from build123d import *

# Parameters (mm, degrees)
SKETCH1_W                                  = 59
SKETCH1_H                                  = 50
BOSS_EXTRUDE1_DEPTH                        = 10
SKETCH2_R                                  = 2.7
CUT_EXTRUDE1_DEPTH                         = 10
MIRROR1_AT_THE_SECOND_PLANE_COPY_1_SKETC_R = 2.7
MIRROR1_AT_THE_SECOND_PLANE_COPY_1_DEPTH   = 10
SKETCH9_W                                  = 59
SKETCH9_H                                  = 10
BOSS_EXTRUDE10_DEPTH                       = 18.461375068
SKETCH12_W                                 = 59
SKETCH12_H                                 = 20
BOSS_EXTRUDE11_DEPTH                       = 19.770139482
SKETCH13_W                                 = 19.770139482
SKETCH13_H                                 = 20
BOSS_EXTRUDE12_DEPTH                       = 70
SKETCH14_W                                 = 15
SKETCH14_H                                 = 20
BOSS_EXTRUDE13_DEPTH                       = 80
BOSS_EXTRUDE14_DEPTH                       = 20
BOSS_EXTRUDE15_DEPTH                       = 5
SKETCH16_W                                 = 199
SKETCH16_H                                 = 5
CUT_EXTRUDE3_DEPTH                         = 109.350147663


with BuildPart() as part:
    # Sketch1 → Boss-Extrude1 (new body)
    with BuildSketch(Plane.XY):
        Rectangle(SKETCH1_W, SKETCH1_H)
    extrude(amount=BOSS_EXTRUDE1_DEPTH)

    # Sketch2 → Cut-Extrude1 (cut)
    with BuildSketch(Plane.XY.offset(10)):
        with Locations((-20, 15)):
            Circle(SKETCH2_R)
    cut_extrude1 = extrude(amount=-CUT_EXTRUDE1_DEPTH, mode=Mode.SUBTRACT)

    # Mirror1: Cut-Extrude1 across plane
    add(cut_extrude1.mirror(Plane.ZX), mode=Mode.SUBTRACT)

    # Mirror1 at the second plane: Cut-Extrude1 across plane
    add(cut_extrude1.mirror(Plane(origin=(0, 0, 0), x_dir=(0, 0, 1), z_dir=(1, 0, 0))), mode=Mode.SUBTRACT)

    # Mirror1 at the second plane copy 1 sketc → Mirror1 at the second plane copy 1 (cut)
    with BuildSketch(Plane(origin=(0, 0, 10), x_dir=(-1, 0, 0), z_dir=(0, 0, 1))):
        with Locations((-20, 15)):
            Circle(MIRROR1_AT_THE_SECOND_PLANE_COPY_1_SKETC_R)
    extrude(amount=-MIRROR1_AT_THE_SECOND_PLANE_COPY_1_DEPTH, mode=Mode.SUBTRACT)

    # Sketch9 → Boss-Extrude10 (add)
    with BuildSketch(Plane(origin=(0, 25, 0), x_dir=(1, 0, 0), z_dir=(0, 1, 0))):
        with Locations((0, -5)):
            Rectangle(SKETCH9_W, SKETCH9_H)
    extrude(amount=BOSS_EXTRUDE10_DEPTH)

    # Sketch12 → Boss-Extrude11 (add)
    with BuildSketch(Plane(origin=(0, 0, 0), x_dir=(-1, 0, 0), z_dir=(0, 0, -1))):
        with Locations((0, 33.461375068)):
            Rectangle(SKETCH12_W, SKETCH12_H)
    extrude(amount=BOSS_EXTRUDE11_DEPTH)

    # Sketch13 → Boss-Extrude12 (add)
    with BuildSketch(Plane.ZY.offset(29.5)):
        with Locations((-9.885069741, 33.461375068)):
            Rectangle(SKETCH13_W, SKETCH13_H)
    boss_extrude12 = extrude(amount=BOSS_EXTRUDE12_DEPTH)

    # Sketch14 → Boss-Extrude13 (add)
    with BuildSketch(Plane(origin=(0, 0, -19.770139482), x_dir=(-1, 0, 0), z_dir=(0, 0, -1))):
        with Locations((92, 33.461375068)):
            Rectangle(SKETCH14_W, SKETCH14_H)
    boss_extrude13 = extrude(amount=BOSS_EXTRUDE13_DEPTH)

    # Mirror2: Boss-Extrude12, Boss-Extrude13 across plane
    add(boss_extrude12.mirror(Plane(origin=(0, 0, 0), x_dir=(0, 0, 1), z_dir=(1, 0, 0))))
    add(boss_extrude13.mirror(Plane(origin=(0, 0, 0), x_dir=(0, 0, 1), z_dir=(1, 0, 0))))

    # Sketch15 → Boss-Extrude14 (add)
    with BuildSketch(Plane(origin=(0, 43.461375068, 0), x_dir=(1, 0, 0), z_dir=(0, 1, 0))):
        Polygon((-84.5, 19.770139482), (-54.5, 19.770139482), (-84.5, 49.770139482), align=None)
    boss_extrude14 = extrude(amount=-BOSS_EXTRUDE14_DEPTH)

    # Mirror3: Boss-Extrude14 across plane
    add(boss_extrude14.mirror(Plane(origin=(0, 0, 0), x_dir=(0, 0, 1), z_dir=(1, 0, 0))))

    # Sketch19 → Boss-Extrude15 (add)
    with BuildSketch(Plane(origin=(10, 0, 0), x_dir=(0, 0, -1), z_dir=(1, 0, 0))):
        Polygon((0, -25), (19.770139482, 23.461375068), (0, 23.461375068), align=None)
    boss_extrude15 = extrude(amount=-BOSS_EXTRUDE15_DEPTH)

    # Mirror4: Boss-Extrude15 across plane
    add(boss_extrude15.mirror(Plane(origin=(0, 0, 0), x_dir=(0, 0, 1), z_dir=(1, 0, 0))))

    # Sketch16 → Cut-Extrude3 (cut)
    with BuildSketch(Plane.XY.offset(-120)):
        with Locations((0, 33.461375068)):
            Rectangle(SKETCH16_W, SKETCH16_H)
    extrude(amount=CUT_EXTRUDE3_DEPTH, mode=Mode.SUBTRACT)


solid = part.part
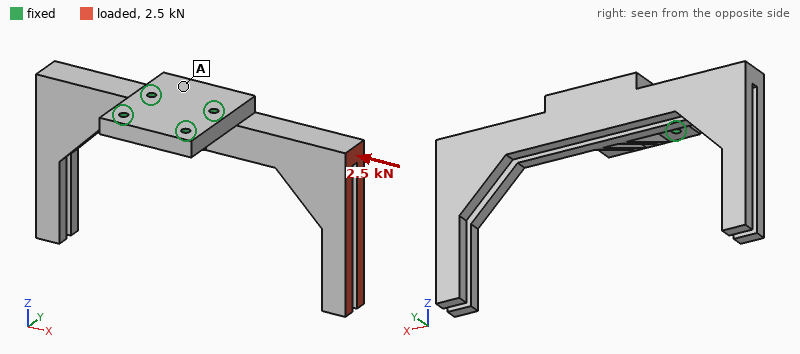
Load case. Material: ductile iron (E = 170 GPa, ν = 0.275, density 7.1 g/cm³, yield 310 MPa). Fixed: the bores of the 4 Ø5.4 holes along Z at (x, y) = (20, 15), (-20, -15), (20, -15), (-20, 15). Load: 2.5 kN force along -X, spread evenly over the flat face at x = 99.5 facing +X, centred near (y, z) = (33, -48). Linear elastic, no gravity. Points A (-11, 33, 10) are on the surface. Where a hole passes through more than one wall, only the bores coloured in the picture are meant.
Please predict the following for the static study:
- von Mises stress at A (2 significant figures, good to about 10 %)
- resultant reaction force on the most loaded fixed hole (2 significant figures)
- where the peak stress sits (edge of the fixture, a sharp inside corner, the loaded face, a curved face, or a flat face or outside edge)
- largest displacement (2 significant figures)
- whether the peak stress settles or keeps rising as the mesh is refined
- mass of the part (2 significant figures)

14 MPa
3.7 kN
edge of the fixture
0.38 mm
keeps rising
1.2 kg
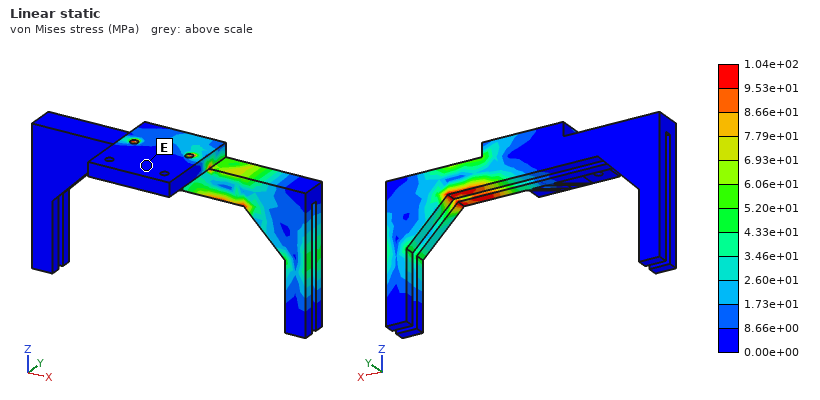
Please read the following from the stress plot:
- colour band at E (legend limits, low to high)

0.00e+00 to 8.66e+00 MPa
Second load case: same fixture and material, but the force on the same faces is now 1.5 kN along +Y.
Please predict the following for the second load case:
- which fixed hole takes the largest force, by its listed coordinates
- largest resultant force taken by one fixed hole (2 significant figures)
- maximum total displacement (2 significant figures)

(20, 15)
3.9 kN
1.1 mm
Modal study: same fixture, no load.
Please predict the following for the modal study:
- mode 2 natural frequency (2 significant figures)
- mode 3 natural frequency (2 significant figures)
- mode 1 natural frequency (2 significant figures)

570 Hz
820 Hz
560 Hz
